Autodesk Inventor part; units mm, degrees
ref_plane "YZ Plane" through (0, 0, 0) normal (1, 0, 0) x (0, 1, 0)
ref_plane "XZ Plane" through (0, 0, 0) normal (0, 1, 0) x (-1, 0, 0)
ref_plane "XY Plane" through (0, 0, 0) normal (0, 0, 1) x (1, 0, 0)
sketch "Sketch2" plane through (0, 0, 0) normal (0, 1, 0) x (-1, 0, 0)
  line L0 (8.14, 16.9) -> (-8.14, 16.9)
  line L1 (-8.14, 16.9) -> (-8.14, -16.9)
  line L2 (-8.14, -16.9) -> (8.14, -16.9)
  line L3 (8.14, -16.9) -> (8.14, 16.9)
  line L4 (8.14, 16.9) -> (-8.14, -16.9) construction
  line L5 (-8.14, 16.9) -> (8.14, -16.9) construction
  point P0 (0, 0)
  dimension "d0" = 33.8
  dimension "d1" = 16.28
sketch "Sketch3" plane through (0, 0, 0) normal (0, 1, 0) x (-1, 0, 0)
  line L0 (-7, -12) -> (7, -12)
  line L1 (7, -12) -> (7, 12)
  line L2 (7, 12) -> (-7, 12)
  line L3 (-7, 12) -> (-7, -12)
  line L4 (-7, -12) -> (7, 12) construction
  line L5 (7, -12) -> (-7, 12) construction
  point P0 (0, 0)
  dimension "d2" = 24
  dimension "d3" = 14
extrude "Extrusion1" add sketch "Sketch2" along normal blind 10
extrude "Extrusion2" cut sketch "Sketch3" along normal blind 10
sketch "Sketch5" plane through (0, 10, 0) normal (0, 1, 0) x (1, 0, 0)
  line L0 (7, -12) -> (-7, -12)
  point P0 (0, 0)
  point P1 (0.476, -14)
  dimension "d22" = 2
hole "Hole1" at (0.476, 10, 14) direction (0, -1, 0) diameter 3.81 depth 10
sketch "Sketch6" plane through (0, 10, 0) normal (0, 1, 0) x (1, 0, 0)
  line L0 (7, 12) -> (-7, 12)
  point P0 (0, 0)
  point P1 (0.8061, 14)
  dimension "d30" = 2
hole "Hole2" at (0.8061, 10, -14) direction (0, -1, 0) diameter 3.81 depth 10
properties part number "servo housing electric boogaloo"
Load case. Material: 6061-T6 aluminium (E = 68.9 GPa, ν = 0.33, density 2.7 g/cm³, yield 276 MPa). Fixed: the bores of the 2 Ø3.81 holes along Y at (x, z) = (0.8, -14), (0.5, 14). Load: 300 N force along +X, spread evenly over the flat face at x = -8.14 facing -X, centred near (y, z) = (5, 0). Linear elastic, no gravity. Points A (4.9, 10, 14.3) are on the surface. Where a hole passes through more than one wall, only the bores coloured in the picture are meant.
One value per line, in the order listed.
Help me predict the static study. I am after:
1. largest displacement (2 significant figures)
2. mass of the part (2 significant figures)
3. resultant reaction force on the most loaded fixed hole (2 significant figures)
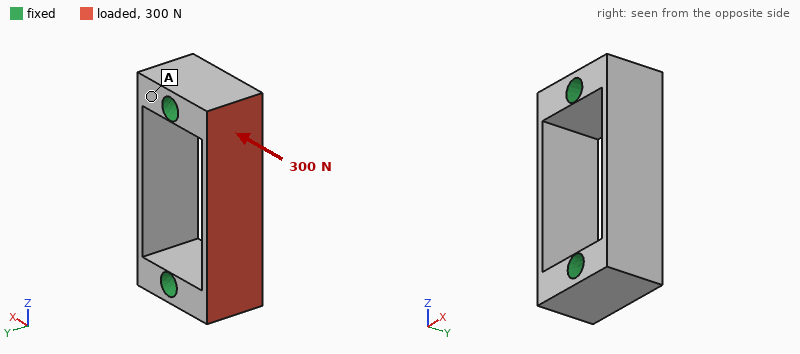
0.11 mm
5.2 g
170 N
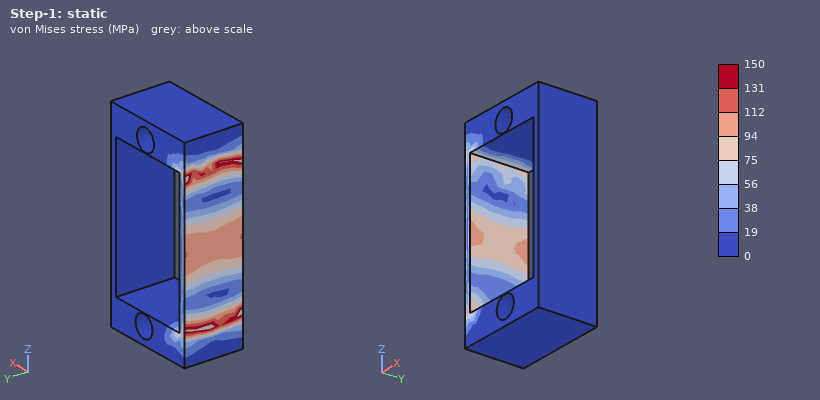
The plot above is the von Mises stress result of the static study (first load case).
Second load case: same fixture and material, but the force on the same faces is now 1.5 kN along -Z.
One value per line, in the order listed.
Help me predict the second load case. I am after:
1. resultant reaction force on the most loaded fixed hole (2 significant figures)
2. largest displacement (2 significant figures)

780 N
26 µm
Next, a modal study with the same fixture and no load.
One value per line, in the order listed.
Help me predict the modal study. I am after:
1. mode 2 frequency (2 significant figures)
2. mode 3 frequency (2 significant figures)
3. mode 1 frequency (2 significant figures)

9500 Hz
17 kHz
9500 Hz
